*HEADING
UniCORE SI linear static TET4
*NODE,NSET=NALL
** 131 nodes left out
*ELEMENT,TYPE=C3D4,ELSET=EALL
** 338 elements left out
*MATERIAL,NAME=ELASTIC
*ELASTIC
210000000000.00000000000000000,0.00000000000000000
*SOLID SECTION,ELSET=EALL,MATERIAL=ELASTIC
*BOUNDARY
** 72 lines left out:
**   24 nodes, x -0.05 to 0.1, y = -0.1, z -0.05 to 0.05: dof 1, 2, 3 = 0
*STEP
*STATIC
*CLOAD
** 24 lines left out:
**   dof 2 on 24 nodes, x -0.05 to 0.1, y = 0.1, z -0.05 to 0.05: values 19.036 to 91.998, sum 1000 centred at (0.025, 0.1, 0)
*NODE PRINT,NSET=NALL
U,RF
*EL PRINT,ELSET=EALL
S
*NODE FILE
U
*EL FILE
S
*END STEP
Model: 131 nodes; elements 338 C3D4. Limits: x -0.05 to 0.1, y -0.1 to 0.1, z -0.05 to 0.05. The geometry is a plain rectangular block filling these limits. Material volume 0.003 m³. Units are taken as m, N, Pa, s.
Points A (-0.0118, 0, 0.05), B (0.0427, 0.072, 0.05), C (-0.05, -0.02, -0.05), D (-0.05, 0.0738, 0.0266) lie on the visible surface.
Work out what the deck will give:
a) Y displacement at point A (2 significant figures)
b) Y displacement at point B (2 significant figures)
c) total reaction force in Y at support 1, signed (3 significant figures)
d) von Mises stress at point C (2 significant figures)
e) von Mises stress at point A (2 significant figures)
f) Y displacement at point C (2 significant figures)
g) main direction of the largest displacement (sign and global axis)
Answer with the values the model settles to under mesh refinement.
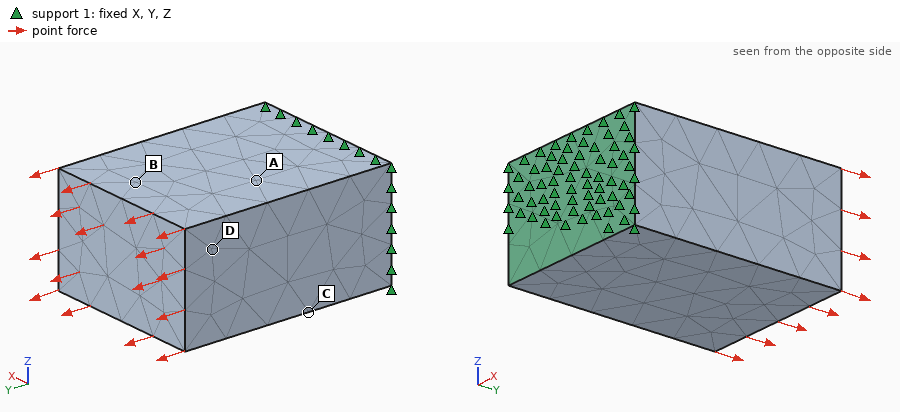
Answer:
3.2e-08 m
5.5e-08 m
-1000 N
67000 Pa
66000 Pa
2.5e-08 m
+Y
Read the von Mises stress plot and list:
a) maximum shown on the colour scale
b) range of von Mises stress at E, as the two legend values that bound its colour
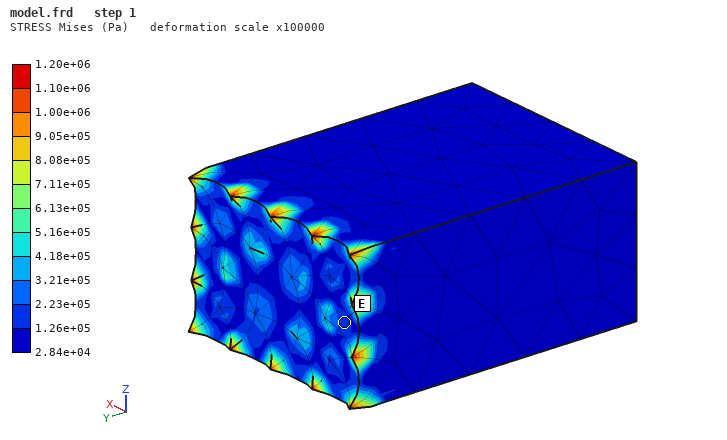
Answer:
1.20e+06 Pa
1.26e+05 to 2.23e+05 Pa
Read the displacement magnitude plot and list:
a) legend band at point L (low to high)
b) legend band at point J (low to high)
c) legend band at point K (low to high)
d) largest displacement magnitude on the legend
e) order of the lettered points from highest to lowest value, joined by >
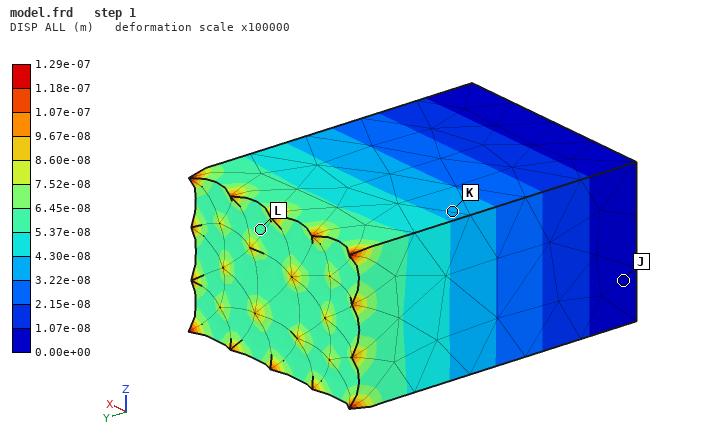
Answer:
5.37e-08 to 6.45e-08 m
0.00e+00 to 1.07e-08 m
3.22e-08 to 4.30e-08 m
1.29e-07 m
L > K > J
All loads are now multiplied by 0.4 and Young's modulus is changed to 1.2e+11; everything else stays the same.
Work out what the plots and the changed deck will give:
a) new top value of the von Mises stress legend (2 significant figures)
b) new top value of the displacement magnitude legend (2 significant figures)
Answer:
4.8e+05 Pa
9.0e-08 m
